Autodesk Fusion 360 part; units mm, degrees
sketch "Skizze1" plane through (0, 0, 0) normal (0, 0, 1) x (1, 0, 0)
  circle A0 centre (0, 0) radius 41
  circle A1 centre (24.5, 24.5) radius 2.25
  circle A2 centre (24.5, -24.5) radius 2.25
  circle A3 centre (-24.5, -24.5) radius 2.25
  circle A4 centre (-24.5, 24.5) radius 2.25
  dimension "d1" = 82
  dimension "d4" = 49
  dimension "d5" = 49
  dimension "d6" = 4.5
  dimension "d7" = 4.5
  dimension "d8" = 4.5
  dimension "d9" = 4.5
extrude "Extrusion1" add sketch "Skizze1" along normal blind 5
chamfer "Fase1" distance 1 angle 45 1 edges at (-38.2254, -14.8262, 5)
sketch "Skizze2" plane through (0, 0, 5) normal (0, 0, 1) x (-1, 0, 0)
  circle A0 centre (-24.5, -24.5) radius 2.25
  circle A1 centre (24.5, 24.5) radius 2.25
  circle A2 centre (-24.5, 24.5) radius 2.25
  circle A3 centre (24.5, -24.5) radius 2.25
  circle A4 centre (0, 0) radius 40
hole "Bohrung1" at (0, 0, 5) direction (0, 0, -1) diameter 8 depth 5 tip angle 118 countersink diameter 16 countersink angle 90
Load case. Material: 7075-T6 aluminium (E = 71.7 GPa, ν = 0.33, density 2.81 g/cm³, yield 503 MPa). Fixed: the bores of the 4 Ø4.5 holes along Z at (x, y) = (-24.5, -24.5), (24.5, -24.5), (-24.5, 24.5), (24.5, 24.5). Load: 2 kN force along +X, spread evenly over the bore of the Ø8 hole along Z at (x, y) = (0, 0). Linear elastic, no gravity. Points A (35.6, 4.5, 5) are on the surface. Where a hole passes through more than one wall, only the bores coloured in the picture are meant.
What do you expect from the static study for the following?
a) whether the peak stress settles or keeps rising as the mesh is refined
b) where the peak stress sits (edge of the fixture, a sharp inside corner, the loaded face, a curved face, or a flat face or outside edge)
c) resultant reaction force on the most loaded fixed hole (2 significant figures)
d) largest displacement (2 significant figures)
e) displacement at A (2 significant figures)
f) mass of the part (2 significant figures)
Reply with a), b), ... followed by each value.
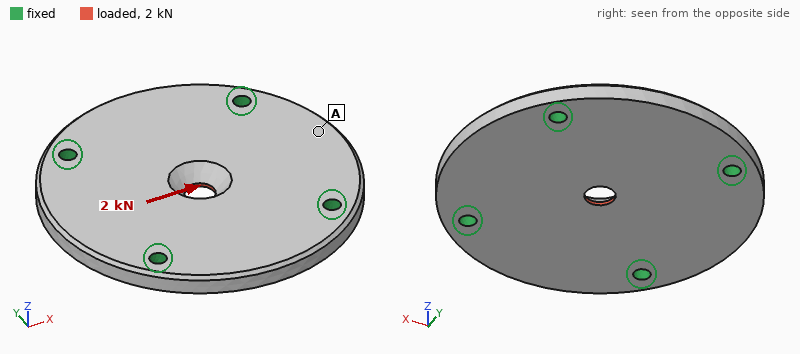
a) keeps rising
b) a sharp inside corner
c) 520 N
d) 8.7 µm
e) 2.4 µm
f) 71 g
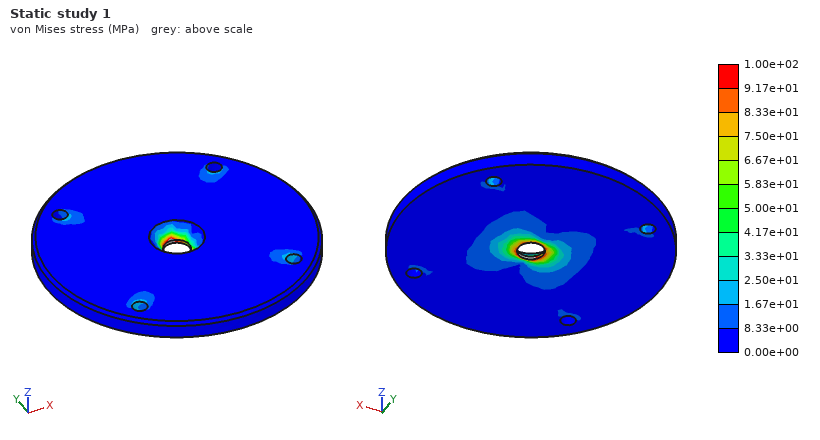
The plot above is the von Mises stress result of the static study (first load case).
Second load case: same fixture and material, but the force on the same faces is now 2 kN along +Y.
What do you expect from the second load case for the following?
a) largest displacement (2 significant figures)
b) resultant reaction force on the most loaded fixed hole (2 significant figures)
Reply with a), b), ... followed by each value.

a) 8.7 µm
b) 520 N
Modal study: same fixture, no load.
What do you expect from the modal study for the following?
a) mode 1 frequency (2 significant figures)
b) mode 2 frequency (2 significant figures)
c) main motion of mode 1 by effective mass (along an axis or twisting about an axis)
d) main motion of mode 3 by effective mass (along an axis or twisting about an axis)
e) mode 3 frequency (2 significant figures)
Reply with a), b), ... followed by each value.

a) 7500 Hz
b) 8200 Hz
c) along Z
d) twisting about Y
e) 8700 Hz
